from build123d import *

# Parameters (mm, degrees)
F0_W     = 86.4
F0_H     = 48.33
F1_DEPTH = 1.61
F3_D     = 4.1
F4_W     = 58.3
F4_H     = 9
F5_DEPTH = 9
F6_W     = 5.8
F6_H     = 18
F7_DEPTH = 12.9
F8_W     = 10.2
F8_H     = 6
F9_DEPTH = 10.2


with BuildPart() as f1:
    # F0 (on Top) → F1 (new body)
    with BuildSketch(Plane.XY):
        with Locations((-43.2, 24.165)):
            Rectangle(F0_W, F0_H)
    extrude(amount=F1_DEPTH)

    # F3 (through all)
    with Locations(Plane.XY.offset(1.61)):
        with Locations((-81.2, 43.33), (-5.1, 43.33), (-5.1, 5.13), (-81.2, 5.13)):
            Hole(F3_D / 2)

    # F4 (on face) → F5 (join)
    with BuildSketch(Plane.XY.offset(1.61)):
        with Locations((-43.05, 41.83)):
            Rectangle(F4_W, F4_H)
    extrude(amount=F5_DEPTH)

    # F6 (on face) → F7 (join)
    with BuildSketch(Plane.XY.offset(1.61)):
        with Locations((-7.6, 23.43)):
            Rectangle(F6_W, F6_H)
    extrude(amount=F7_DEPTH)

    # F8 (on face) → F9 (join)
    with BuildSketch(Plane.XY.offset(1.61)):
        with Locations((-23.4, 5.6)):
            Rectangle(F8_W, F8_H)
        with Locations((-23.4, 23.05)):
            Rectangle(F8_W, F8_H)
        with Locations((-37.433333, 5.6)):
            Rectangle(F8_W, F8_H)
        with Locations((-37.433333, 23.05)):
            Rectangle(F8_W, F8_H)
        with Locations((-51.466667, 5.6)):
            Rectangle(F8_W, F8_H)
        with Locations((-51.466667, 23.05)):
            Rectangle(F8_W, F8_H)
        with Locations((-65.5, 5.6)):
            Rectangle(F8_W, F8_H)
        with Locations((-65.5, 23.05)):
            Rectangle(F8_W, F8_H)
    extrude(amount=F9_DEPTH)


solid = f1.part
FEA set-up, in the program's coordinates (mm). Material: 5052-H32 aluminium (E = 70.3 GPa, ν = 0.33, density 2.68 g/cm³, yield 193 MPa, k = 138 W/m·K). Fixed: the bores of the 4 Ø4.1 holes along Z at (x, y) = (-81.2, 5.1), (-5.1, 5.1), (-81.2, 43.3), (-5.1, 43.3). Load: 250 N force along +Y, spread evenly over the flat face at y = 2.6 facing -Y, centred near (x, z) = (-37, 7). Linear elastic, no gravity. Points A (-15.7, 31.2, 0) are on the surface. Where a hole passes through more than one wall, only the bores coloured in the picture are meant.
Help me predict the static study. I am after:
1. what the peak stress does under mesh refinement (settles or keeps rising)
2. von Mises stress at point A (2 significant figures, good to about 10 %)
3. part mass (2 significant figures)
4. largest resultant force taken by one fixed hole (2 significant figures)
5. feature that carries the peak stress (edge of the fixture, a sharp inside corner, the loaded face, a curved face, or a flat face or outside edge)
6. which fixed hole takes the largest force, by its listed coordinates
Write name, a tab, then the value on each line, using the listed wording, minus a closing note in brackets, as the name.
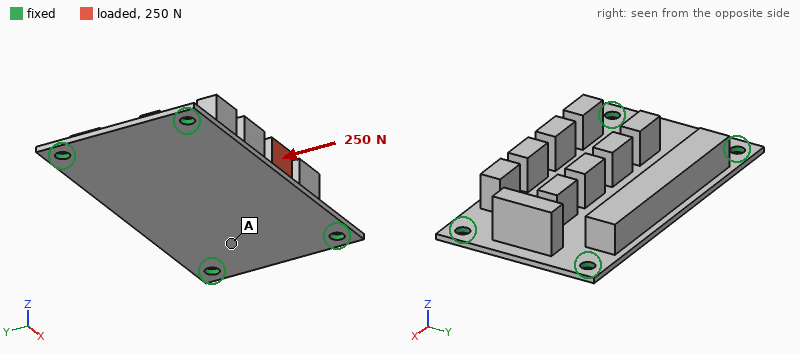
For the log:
what the peak stress does under mesh refinement	keeps rising
von Mises stress at point A	8.6 MPa
part mass	47 g
largest resultant force taken by one fixed hole	110 N
feature that carries the peak stress	edge of the fixture
which fixed hole takes the largest force, by its listed coordinates	(-5.1, 43.3)
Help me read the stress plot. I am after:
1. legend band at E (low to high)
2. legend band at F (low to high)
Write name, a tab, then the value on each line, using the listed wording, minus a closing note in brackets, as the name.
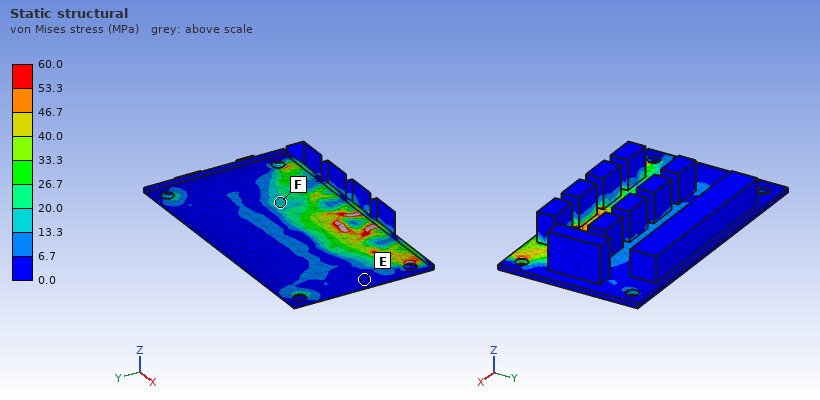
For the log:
legend band at E	0.0 to 6.7 MPa
legend band at F	13.3 to 20.0 MPa
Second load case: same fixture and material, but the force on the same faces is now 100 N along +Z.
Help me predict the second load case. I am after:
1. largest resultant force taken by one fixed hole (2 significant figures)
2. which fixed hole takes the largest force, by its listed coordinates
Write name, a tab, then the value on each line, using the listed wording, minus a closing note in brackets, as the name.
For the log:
largest resultant force taken by one fixed hole	66 N
which fixed hole takes the largest force, by its listed coordinates	(-5.1, 5.1)
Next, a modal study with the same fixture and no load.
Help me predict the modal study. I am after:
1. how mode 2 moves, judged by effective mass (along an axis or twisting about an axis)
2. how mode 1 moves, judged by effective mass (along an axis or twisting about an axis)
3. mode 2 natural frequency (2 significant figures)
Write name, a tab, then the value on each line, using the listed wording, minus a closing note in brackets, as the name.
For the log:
how mode 2 moves, judged by effective mass	along Z
how mode 1 moves, judged by effective mass	along Z
mode 2 natural frequency	2600 Hz
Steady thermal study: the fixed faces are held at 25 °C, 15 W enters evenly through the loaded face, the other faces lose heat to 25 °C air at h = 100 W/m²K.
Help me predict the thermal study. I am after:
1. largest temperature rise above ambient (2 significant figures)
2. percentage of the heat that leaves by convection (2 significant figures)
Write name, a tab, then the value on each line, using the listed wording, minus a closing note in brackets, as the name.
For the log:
largest temperature rise above ambient	39 K
percentage of the heat that leaves by convection	58 %
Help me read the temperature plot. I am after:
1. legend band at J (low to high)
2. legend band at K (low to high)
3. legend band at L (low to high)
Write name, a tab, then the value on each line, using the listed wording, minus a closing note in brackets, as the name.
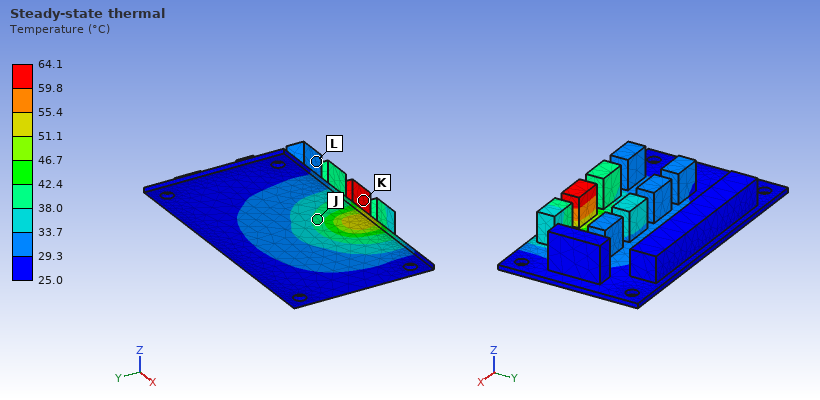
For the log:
legend band at J	38.0 to 42.4 °C
legend band at K	59.8 to 64.1 °C
legend band at L	29.3 to 33.7 °C
